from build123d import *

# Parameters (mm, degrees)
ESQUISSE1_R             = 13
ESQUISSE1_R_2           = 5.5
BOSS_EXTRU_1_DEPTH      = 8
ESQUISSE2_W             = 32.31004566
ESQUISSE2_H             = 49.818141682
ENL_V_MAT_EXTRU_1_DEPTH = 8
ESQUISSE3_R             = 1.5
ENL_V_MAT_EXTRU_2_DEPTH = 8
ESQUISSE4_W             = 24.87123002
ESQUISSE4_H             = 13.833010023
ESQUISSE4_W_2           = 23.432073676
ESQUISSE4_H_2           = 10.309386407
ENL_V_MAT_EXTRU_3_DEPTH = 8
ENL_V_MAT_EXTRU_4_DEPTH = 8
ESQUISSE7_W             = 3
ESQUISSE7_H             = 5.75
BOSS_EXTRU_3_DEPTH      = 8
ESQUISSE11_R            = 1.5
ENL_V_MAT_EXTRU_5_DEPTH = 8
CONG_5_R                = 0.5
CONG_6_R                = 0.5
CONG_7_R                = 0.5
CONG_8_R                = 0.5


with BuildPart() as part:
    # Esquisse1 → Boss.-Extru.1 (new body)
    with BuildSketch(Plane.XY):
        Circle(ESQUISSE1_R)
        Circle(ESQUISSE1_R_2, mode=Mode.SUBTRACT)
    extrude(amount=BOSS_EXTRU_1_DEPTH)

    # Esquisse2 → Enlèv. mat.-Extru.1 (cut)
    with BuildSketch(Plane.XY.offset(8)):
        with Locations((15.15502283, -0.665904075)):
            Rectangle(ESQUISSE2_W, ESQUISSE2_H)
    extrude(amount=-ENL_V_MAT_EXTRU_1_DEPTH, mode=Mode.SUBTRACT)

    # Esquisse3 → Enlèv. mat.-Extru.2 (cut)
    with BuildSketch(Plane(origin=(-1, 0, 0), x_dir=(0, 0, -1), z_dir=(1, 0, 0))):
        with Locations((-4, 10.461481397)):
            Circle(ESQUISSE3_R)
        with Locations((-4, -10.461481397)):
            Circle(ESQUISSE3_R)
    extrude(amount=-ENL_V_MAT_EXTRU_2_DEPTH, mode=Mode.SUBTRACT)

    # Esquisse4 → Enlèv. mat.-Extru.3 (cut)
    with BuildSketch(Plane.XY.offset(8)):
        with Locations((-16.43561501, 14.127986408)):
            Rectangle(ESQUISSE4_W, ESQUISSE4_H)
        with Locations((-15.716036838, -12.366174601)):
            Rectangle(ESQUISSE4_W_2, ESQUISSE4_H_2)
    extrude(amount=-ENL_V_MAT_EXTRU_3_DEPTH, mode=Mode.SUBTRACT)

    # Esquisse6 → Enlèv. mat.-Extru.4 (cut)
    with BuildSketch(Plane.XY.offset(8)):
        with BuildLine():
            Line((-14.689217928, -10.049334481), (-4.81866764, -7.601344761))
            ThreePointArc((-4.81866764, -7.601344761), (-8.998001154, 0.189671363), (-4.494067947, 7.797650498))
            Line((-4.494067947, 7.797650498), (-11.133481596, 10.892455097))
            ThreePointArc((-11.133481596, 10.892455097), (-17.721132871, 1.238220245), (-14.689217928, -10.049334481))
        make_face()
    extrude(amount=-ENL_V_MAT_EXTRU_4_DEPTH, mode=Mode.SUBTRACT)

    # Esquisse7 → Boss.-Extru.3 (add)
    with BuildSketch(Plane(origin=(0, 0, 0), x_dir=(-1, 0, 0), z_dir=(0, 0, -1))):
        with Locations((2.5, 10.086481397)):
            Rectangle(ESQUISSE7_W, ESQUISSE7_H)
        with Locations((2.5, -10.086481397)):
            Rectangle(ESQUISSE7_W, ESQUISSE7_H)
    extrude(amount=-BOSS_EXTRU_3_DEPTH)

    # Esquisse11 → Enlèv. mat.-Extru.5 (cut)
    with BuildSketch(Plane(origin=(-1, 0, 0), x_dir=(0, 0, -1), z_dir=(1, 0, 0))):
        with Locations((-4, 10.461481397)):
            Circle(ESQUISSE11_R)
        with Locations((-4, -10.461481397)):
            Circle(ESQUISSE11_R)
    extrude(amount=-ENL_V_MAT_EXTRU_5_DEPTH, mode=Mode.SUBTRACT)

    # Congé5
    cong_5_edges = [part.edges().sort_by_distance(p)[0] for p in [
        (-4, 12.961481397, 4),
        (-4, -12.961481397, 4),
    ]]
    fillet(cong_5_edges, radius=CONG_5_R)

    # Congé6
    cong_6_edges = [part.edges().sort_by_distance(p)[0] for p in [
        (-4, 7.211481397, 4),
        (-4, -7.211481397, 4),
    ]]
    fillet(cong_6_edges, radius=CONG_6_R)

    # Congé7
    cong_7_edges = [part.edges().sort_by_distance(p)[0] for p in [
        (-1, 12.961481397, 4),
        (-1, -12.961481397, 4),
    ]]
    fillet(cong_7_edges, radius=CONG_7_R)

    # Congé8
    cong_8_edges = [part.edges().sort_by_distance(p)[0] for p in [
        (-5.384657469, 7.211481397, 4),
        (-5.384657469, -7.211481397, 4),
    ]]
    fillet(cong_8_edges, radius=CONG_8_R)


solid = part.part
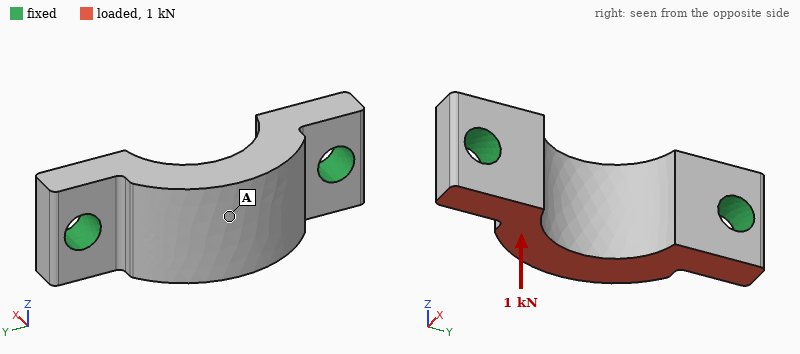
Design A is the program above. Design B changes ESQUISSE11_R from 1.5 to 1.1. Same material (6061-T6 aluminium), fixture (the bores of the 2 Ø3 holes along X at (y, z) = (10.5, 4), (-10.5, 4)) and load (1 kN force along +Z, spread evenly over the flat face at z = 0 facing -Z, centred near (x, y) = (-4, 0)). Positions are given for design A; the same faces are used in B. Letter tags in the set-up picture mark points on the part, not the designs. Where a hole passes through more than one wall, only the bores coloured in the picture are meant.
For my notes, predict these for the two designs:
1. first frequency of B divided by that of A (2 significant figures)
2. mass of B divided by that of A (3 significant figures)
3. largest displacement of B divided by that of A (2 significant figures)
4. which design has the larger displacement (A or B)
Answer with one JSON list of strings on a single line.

["0.87", "1.03", "1.3", "B"]
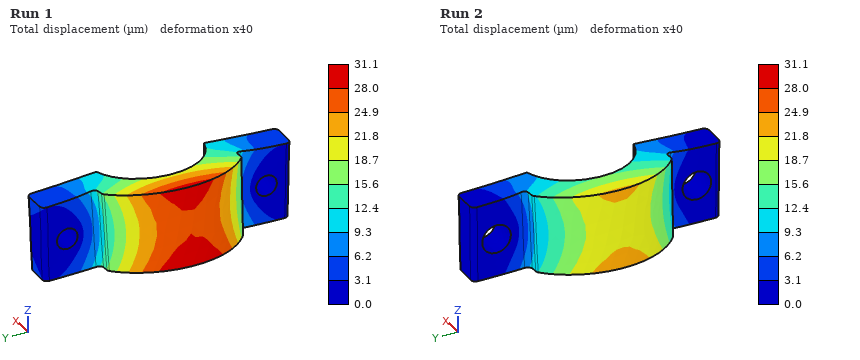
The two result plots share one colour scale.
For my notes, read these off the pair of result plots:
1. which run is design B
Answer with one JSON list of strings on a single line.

["Run 1"]
